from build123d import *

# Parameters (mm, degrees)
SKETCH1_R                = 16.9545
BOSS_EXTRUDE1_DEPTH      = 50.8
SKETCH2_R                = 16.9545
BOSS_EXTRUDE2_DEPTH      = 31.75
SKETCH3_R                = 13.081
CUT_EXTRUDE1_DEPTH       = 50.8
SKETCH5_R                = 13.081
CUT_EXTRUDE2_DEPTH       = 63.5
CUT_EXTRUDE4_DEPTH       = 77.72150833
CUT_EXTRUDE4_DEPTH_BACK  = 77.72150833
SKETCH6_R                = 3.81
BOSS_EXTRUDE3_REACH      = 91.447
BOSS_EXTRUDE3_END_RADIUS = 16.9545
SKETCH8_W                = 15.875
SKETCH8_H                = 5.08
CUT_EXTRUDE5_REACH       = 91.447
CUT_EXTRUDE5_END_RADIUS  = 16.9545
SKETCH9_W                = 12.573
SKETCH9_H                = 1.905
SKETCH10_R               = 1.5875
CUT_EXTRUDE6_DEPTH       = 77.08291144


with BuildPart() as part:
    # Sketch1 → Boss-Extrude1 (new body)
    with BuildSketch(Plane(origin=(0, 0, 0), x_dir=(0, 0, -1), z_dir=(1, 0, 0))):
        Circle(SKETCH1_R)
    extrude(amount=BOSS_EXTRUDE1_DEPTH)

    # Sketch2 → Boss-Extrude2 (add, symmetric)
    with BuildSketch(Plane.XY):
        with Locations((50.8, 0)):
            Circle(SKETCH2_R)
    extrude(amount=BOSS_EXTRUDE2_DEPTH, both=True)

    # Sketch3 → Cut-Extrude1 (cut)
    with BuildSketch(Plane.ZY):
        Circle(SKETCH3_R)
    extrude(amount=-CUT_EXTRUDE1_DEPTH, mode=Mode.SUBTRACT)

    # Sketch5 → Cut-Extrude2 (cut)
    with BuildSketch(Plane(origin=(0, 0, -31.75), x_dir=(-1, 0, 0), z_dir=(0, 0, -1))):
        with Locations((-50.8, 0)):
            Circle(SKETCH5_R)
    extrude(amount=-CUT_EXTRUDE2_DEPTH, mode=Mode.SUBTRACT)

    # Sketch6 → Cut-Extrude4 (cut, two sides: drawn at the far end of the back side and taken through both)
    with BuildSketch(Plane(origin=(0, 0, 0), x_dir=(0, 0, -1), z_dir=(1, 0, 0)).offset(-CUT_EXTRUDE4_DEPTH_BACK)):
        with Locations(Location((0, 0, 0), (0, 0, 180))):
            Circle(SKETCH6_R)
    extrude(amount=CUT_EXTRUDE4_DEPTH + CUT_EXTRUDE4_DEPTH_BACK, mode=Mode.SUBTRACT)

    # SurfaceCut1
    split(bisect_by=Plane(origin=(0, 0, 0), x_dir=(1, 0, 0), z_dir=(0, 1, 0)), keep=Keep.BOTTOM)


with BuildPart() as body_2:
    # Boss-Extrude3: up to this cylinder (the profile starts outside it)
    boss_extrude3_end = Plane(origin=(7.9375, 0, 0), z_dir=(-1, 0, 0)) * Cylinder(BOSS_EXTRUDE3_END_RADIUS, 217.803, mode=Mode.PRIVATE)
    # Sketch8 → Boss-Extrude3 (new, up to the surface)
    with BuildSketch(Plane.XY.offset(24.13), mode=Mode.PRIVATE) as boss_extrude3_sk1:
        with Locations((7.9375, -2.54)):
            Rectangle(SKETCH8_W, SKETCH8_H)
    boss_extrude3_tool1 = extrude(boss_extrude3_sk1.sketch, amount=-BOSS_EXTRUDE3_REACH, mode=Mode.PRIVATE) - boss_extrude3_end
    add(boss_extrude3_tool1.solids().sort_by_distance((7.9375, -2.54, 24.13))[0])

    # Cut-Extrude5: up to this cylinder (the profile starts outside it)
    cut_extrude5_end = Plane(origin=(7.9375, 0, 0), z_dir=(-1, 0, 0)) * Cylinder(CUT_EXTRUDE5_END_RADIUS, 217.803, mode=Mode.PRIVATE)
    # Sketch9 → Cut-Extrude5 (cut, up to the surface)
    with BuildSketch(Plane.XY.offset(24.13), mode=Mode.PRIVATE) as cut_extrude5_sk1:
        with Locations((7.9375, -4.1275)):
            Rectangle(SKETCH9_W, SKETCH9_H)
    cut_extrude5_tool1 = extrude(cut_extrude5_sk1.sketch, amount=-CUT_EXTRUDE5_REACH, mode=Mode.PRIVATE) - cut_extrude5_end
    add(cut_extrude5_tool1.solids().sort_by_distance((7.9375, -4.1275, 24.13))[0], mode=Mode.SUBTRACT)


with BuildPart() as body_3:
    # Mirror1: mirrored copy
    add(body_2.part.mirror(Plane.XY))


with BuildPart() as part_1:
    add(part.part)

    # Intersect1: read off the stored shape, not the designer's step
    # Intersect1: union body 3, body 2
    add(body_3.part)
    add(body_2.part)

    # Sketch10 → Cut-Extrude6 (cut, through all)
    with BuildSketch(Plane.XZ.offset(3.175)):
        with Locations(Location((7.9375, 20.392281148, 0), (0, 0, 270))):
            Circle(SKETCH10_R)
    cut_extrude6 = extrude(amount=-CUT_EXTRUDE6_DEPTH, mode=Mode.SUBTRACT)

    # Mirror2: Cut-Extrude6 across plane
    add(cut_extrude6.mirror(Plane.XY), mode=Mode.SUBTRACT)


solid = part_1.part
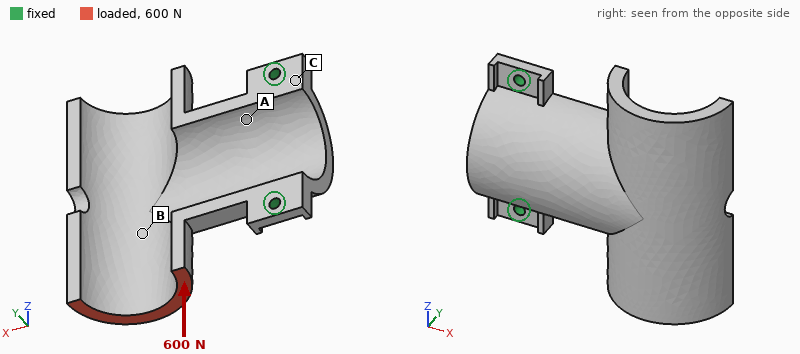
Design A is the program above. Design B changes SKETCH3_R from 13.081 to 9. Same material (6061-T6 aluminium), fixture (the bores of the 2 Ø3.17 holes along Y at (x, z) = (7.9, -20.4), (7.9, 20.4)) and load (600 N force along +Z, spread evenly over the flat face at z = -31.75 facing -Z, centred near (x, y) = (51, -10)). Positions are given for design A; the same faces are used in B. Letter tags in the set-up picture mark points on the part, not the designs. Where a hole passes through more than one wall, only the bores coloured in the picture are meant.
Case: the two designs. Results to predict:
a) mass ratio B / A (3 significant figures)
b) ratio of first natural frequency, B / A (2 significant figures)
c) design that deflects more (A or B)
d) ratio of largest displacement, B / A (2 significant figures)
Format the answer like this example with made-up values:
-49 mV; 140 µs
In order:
1.32; 1.0; A; 0.34
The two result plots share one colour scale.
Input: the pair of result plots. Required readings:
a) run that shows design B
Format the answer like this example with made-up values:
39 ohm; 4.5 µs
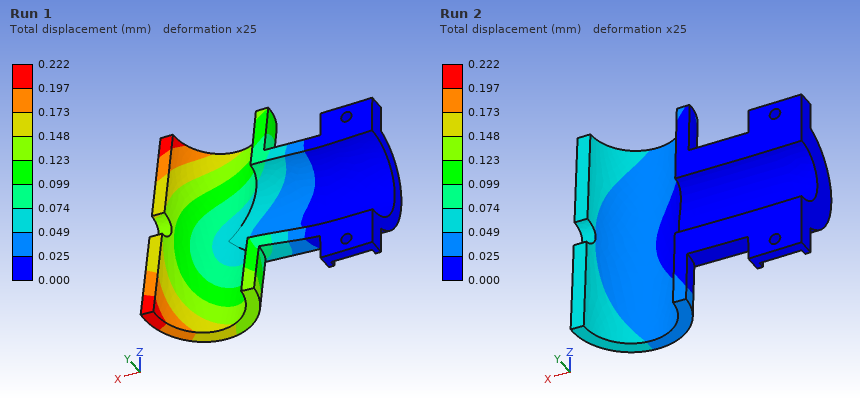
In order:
Run 2
